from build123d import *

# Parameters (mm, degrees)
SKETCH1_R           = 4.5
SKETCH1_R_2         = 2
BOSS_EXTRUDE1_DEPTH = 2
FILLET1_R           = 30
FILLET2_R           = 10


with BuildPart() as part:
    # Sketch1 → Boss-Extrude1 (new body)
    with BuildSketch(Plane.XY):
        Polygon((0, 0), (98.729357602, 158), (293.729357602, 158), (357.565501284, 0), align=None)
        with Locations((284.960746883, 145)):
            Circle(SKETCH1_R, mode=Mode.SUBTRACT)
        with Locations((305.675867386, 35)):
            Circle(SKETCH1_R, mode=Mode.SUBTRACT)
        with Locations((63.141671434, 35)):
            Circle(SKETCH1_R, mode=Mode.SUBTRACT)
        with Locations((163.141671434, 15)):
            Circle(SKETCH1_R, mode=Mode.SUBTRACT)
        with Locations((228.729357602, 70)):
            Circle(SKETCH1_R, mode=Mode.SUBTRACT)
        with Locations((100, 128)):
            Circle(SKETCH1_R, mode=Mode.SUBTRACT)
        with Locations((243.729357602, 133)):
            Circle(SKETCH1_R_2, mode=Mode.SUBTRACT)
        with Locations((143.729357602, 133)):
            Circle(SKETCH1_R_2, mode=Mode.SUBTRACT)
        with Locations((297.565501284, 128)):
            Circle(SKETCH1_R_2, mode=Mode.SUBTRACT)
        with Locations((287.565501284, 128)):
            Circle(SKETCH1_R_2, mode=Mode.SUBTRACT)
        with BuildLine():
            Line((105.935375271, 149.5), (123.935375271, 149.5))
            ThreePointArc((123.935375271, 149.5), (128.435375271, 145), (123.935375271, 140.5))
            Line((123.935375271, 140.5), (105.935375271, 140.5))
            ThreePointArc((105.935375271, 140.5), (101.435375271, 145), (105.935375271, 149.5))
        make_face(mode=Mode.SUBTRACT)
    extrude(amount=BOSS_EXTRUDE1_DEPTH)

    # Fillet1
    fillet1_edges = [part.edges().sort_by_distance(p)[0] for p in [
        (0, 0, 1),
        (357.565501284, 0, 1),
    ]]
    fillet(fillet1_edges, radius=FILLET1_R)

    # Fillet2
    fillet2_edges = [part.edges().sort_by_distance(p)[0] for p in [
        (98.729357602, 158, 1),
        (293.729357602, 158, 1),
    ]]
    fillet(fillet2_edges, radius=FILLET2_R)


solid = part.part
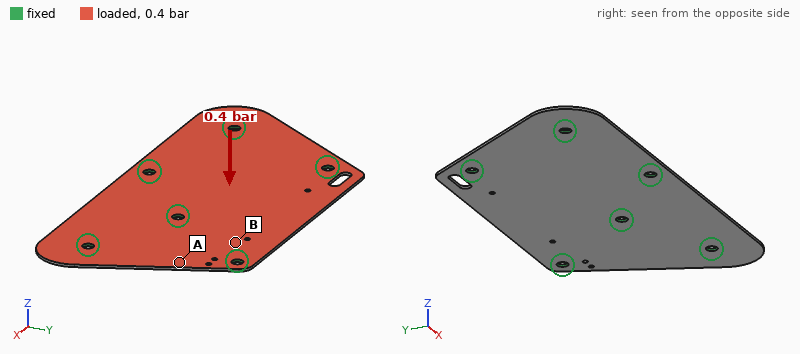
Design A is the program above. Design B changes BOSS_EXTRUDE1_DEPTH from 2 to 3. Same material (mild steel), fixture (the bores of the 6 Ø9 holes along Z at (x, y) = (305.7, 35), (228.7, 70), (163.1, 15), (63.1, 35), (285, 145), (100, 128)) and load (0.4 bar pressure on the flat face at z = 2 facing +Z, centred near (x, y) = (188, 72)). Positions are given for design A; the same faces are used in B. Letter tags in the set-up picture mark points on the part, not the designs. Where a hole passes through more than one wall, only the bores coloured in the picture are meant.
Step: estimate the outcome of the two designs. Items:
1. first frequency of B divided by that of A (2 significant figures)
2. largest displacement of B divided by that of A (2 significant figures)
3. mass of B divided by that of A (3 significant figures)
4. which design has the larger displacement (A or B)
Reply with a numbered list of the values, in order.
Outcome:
1. 1.5
2. 0.30
3. 1.50
4. A
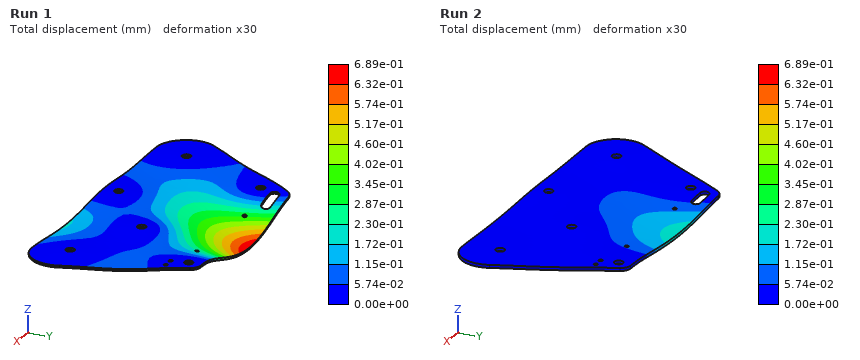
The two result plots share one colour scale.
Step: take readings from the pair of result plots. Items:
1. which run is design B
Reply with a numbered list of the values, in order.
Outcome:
1. Run 2
